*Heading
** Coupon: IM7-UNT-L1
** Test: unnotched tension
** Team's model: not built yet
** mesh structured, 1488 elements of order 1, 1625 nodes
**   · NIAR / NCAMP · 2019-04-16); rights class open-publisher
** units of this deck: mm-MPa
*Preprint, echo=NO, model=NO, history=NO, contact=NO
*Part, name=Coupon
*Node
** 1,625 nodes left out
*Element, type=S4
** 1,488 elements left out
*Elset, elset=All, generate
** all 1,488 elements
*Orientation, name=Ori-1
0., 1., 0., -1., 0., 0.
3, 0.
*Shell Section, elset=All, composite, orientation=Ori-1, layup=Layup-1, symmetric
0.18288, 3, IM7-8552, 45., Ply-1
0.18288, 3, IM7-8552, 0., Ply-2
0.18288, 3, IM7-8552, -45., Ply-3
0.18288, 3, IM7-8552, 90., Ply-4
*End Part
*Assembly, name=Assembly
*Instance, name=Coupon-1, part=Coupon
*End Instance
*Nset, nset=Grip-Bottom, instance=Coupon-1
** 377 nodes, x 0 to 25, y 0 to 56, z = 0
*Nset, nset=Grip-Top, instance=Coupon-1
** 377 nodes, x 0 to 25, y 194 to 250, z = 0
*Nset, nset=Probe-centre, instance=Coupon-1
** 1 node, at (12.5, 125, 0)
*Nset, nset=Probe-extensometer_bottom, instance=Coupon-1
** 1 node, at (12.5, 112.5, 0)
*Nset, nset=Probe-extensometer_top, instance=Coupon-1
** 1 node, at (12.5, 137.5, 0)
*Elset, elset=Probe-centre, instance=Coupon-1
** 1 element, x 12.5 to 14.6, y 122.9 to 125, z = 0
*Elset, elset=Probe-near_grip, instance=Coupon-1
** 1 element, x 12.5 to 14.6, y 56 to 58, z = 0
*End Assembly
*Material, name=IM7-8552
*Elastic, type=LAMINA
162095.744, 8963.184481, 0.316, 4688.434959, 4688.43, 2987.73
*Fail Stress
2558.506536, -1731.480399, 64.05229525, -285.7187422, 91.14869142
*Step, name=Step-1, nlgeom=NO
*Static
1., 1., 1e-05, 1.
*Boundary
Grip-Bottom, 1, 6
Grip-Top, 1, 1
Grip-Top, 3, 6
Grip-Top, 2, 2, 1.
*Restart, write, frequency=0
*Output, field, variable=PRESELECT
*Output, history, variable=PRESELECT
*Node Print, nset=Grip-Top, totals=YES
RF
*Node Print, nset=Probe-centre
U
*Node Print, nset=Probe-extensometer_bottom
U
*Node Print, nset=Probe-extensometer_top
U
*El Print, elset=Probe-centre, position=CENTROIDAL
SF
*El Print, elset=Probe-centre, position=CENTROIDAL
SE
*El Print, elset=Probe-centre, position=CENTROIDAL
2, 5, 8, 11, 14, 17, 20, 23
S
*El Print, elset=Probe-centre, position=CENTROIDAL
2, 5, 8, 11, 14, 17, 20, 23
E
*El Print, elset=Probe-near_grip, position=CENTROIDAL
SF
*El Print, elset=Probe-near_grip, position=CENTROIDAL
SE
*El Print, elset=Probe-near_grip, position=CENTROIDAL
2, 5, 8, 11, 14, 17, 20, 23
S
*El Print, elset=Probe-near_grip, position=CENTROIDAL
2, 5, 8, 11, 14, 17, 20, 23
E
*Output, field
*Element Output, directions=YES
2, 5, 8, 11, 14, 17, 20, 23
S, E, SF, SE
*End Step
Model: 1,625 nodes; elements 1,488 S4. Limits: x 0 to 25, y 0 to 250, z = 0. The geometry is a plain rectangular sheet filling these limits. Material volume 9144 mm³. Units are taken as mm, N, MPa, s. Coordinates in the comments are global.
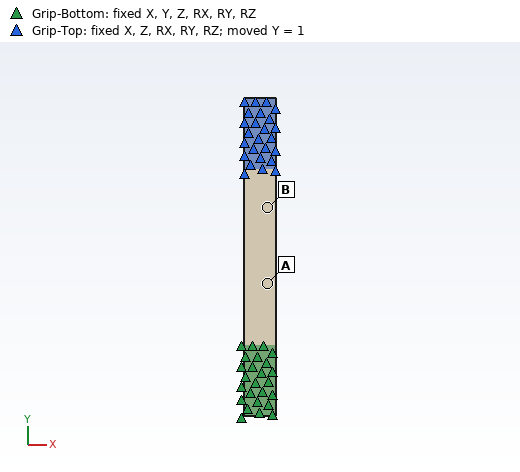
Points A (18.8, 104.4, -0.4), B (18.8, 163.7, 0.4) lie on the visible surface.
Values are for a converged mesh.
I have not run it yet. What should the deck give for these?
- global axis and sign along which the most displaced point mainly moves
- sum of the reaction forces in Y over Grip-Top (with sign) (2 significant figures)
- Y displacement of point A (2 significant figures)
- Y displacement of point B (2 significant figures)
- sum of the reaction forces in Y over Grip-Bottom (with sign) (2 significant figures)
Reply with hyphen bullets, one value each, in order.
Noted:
- +Y
- 16000 N
- 0.35 mm
- 0.78 mm
- -16000 N
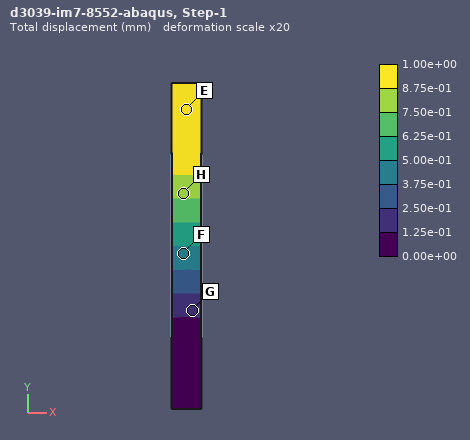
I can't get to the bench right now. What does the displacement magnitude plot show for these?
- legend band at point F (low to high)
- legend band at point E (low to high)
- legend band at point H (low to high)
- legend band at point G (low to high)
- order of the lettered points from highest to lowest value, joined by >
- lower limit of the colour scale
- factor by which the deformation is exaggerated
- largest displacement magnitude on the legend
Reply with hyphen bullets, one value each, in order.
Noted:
- 3.75e-01 to 5.00e-01 mm
- 8.75e-01 to 1.00e+00 mm
- 7.50e-01 to 8.75e-01 mm
- 1.25e-01 to 2.50e-01 mm
- E > H > F > G
- 0.00e+00 mm
- 20
- 1.00e+00 mm
